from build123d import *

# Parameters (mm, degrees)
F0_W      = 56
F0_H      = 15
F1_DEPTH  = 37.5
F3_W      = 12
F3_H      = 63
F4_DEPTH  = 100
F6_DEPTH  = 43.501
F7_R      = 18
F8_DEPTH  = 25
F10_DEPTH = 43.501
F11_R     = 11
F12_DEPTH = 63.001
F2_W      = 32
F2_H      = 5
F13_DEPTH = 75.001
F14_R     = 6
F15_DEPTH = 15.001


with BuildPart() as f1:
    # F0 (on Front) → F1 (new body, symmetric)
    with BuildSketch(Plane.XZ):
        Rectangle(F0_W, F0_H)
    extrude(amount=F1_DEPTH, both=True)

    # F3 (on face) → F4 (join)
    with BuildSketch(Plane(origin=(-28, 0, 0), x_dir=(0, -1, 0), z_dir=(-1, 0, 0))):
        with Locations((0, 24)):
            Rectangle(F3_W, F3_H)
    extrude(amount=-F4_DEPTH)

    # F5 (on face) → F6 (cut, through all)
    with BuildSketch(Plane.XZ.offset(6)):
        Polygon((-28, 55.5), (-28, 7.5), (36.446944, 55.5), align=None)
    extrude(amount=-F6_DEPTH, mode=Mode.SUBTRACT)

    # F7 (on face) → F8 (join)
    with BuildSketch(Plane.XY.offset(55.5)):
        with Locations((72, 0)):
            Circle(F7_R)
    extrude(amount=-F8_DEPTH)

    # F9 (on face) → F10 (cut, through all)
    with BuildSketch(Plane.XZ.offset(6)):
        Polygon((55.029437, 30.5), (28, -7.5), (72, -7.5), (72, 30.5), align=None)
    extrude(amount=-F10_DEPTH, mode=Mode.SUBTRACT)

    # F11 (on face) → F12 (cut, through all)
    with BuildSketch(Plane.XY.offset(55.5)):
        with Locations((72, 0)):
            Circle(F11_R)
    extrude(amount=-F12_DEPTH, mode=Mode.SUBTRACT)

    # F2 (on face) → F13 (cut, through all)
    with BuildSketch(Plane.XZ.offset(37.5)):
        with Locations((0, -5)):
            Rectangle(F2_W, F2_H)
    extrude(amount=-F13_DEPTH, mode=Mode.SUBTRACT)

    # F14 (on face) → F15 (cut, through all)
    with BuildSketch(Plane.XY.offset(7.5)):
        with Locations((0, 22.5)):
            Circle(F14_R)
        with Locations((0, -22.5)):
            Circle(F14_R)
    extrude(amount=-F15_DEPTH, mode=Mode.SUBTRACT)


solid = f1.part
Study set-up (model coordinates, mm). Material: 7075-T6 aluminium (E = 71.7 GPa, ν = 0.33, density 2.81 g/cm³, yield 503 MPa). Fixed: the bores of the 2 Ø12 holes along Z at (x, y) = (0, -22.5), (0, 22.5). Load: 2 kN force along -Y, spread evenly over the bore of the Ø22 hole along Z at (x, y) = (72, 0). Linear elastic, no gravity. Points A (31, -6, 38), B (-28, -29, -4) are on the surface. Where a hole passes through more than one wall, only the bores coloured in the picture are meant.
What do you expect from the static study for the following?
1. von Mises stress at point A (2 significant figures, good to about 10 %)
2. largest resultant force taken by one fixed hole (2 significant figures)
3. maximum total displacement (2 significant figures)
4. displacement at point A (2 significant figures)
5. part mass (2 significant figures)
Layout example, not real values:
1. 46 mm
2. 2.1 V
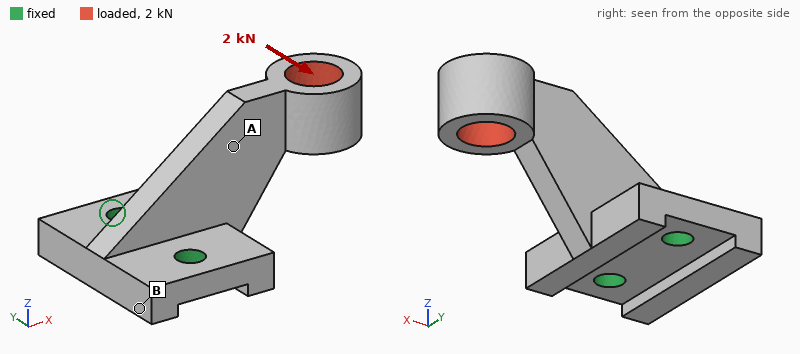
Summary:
1. 81 MPa
2. 3.7 kN
3. 0.90 mm
4. 0.18 mm
5. 260 g
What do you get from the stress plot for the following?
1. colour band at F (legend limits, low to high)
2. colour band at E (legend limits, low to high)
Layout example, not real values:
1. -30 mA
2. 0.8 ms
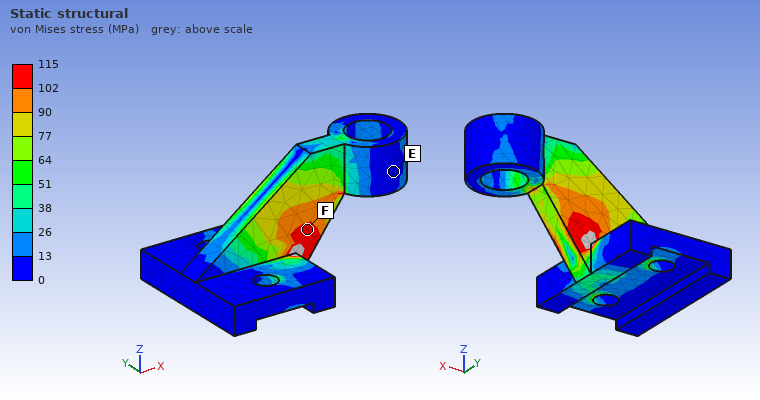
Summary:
1. 102 to 115 MPa
2. 0 to 13 MPa
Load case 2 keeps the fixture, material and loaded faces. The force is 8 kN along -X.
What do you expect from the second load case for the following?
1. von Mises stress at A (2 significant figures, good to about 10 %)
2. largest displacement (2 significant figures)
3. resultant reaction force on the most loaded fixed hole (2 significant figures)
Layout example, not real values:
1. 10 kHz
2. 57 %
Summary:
1. 38 MPa
2. 0.60 mm
3. 4.1 kN
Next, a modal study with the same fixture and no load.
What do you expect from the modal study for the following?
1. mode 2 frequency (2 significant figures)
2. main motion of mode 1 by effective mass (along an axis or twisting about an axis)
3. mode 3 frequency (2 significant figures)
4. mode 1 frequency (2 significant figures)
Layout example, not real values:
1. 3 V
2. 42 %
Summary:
1. 1800 Hz
2. along Y
3. 3600 Hz
4. 1200 Hz
